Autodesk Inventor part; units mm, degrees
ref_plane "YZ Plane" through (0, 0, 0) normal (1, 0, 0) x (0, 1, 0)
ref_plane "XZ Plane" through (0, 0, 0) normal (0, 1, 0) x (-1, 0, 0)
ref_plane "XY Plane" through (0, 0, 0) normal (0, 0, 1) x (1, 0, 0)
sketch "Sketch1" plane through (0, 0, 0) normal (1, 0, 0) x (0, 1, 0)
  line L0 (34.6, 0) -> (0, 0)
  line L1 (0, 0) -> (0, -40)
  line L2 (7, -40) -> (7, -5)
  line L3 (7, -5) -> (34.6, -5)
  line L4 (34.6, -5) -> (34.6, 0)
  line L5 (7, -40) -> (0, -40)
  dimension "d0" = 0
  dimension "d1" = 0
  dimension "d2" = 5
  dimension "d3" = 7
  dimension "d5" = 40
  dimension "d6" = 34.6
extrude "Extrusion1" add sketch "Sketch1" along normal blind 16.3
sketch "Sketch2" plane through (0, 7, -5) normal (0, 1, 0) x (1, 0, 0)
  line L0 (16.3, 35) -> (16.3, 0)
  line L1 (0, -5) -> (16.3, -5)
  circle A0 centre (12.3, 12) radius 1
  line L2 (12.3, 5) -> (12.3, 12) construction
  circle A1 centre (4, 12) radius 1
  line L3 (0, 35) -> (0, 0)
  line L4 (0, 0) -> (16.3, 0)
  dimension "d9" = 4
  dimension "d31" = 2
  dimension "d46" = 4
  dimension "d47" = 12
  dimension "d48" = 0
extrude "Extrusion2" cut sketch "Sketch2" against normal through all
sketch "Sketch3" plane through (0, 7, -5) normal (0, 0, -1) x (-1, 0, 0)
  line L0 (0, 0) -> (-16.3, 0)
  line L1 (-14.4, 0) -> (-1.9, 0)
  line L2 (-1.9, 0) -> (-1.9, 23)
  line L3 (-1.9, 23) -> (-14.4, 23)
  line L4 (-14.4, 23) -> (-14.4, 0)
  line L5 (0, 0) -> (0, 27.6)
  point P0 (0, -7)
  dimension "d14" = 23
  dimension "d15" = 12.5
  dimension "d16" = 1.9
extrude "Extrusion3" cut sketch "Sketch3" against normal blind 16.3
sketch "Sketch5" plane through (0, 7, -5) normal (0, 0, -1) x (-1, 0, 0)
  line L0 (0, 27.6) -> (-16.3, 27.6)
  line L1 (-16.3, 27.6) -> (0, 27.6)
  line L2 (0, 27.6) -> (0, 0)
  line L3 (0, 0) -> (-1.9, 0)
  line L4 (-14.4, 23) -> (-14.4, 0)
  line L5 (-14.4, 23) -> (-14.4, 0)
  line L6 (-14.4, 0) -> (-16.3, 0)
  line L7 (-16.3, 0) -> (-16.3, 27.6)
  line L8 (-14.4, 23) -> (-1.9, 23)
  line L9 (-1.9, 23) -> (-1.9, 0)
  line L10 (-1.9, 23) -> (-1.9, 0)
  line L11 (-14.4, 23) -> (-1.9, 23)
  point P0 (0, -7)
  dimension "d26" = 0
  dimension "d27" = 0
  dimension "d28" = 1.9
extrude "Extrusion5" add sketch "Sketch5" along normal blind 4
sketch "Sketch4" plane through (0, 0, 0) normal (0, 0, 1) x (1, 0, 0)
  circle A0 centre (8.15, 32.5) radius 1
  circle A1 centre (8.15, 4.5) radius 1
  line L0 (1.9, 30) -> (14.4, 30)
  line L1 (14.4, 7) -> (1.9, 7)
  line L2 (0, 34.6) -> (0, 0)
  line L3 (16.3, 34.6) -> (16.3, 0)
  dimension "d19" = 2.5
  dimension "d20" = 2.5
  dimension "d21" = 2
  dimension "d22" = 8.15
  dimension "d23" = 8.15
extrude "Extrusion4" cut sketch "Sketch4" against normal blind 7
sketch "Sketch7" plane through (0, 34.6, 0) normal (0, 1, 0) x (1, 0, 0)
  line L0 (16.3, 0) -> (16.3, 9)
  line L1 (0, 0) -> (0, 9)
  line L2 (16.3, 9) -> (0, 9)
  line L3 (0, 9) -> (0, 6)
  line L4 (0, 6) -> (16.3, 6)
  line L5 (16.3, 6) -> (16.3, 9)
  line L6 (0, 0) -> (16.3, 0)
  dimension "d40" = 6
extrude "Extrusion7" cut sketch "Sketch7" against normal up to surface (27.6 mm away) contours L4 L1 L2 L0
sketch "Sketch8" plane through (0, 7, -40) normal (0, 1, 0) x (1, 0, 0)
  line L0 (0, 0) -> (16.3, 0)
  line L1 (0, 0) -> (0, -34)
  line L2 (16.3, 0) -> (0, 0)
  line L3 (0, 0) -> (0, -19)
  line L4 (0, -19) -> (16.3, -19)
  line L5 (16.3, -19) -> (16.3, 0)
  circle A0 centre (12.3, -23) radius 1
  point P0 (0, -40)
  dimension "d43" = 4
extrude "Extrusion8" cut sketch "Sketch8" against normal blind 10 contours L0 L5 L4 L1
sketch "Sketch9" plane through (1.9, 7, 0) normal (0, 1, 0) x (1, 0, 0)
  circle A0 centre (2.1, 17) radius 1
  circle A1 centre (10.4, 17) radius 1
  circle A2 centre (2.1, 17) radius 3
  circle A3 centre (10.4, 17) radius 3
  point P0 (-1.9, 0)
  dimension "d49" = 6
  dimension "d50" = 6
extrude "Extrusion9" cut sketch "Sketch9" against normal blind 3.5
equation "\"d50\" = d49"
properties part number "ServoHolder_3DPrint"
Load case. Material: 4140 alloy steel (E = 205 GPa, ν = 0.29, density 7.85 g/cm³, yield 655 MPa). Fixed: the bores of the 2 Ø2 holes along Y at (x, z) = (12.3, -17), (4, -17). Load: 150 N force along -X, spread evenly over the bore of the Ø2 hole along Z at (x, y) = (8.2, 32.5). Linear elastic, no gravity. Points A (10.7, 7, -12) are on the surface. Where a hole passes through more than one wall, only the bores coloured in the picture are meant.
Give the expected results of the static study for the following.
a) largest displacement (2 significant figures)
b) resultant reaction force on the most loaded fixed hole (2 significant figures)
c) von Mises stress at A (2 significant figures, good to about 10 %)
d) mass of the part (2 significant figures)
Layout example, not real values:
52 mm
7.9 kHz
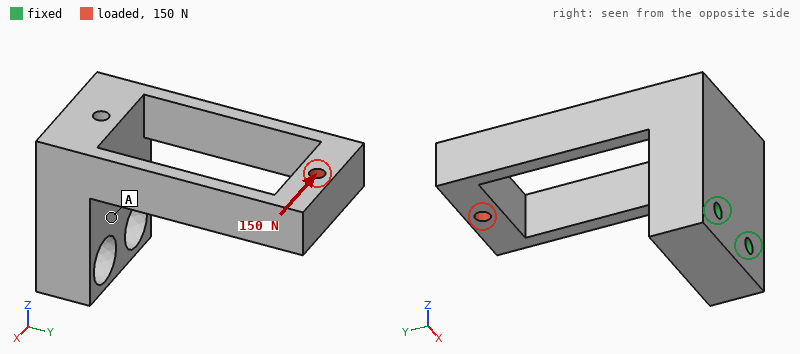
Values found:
0.16 mm
490 N
36 MPa
24 g
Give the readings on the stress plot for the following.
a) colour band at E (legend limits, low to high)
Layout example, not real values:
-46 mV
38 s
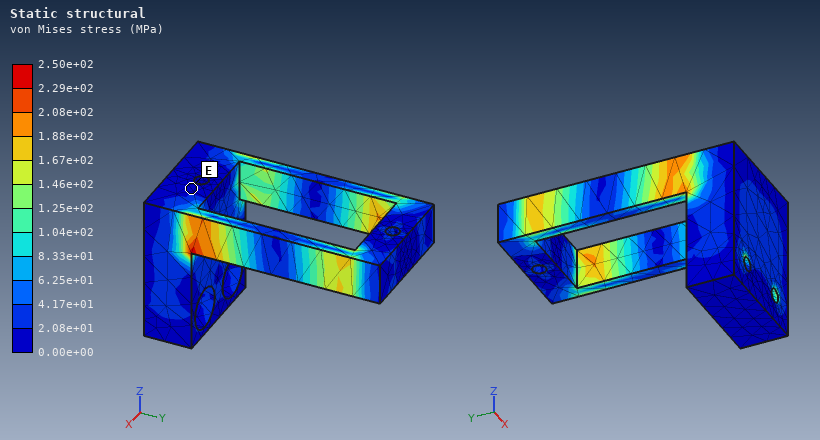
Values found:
0.00e+00 to 2.08e+01 MPa
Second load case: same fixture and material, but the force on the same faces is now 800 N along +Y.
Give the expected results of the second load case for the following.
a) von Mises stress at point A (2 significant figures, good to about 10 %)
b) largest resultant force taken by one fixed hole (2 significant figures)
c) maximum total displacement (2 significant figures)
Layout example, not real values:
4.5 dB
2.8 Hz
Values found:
52 MPa
400 N
93 µm
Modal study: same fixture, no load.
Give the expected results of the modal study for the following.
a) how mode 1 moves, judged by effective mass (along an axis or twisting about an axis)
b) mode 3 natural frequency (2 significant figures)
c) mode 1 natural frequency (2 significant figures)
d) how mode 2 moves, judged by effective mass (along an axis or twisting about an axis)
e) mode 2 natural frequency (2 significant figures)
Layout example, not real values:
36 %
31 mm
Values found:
along X
7300 Hz
2200 Hz
along Z
2700 Hz
